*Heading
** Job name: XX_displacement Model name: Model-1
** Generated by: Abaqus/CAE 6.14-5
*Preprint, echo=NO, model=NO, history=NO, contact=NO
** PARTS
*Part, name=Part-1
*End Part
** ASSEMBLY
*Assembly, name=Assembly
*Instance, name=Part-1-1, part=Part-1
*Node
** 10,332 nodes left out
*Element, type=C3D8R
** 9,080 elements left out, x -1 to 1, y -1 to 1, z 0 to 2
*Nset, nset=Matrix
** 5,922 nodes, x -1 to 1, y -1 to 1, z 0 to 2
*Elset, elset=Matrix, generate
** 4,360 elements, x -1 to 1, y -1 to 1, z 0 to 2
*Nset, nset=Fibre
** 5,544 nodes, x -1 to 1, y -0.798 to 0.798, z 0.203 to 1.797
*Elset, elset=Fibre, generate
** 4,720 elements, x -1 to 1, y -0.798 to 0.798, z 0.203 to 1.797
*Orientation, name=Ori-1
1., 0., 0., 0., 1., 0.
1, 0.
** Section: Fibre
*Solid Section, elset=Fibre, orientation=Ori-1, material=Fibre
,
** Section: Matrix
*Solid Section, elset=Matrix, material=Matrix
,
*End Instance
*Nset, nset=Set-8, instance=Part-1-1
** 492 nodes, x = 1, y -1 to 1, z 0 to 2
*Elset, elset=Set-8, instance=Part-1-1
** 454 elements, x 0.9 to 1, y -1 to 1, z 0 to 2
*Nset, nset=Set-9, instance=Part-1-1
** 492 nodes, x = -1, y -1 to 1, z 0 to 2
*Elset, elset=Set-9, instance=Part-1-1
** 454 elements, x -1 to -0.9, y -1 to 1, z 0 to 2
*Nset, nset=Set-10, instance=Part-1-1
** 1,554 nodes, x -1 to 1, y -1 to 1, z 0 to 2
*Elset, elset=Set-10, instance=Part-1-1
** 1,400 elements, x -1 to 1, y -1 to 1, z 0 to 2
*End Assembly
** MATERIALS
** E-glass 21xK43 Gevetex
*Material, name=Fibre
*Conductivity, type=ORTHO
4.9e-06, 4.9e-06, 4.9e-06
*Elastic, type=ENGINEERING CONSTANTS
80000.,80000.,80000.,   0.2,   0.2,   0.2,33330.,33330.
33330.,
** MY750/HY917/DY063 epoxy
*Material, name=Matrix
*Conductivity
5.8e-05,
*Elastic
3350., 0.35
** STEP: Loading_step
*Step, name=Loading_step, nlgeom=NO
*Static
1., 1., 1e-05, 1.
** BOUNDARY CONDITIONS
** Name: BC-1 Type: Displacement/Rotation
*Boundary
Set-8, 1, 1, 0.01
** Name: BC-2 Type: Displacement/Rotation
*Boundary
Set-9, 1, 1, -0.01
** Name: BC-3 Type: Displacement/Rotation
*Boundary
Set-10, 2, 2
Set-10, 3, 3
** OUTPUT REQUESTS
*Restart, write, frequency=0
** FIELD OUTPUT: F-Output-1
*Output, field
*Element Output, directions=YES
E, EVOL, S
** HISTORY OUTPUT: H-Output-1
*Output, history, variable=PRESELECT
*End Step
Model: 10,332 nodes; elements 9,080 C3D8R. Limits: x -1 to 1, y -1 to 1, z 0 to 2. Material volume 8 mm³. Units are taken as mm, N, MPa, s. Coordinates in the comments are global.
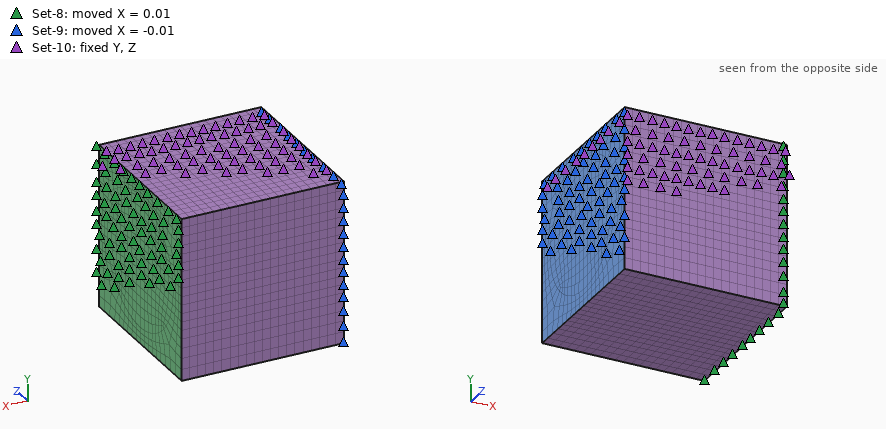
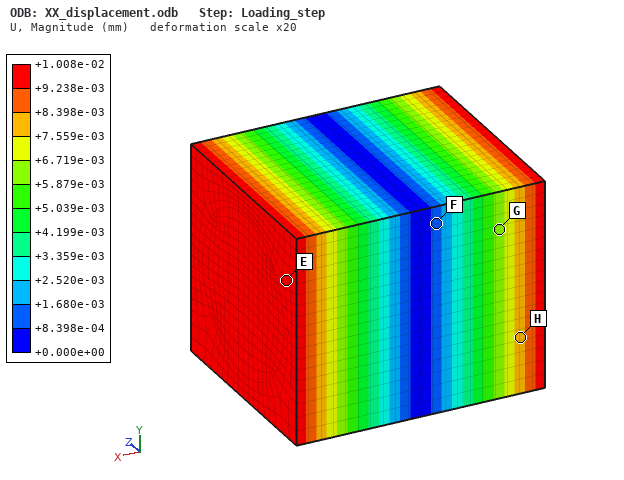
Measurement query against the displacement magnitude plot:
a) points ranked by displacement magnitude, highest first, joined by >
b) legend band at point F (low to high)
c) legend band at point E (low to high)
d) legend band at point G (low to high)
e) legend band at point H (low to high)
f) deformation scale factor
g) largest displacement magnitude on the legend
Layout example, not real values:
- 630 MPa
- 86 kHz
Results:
- E > H > G > F
- +8.398e-04 to +1.680e-03 mm
- +9.238e-03 to +1.008e-02 mm
- +5.879e-03 to +6.719e-03 mm
- +7.559e-03 to +8.398e-03 mm
- 20
- +1.008e-02 mm
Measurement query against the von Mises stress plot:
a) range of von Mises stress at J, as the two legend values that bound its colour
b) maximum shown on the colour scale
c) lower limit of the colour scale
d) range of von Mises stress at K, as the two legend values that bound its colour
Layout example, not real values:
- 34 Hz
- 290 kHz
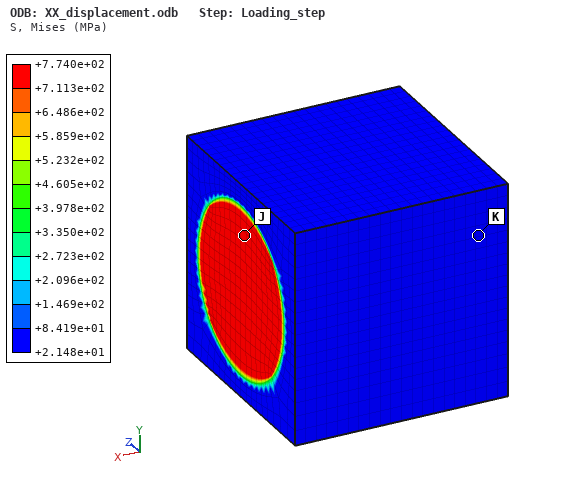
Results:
- +7.113e+02 to +7.740e+02 MPa
- +7.740e+02 MPa
- +2.148e+01 MPa
- +2.148e+01 to +8.419e+01 MPa
